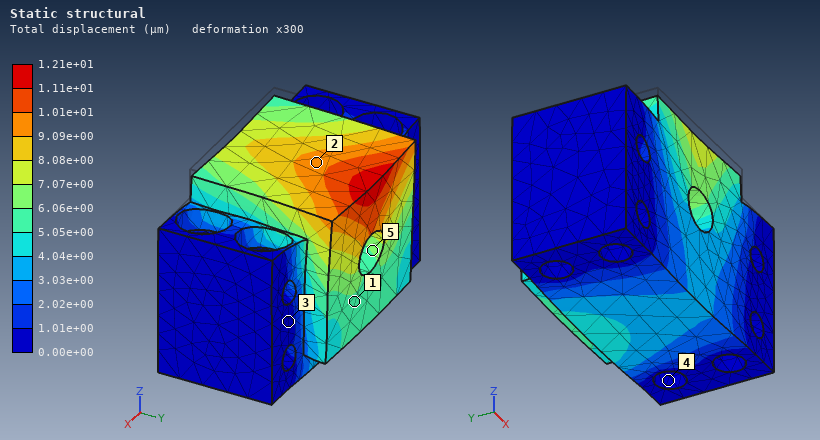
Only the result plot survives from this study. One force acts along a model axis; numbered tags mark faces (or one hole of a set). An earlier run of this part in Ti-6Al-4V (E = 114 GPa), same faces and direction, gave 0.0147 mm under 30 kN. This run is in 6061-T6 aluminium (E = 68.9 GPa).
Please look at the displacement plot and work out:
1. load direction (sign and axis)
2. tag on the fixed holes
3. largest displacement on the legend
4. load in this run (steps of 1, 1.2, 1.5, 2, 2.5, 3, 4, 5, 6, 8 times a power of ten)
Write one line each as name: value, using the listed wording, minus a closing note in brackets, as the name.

load direction: -Z
tag on the fixed holes: 4
largest displacement on the legend: 1.21e+01 µm
load in this run: 15 kN
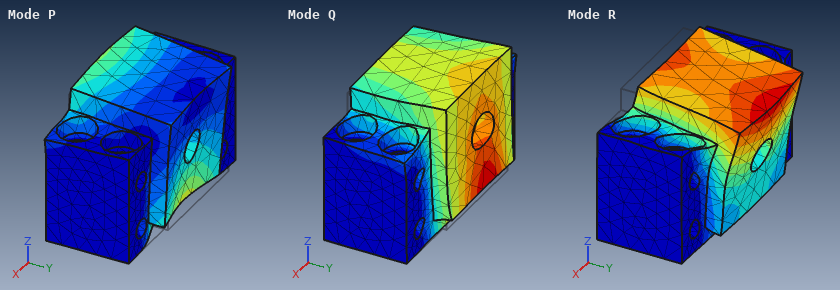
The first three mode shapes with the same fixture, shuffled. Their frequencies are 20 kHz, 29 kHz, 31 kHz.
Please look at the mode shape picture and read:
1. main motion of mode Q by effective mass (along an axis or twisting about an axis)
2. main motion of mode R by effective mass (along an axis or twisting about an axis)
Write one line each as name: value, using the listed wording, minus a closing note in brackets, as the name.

main motion of mode Q by effective mass: along Z
main motion of mode R by effective mass: along Y
